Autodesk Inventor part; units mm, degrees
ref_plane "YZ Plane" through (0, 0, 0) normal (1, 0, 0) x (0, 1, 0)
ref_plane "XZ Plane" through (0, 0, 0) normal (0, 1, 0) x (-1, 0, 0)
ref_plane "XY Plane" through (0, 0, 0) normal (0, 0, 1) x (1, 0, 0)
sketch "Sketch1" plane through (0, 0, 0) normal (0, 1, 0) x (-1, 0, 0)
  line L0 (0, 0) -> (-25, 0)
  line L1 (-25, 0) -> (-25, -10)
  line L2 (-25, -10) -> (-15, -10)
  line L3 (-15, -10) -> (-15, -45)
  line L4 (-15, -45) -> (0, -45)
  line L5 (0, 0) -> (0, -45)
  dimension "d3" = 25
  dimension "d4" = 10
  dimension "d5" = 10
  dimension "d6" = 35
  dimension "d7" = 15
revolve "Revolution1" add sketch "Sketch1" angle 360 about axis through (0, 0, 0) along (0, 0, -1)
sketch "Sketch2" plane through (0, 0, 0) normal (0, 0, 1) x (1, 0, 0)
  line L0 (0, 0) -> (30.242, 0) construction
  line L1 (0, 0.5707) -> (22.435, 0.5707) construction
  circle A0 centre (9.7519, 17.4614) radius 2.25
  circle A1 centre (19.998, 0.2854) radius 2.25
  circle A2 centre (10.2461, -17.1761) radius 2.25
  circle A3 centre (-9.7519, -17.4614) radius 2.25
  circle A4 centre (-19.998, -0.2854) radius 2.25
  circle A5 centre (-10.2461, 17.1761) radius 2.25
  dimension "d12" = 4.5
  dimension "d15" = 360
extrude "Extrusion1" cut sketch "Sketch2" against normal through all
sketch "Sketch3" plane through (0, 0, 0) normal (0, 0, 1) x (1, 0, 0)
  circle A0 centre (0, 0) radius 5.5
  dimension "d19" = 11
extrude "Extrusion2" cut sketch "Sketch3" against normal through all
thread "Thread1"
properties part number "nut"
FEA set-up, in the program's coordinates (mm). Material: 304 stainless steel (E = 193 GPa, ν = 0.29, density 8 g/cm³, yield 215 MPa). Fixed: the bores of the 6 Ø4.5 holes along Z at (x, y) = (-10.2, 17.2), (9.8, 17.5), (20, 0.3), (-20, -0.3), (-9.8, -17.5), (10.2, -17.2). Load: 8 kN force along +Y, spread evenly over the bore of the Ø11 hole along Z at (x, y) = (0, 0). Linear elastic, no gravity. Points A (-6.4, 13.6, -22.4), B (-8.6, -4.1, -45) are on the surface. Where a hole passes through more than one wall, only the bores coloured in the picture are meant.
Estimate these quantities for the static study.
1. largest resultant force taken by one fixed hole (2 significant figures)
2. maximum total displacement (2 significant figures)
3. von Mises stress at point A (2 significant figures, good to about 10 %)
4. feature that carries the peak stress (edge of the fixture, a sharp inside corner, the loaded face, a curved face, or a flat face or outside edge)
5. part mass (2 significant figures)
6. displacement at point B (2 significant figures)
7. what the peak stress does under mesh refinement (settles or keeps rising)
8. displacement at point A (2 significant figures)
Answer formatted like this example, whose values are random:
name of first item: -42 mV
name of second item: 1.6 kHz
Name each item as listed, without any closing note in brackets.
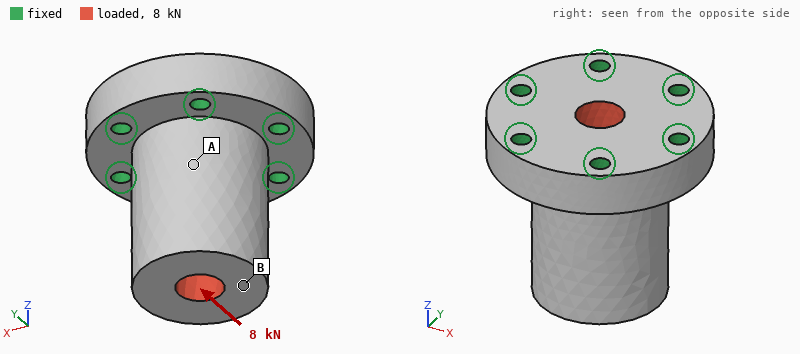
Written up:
largest resultant force taken by one fixed hole: 2.8 kN
maximum total displacement: 14 µm
von Mises stress at point A: 16 MPa
feature that carries the peak stress: edge of the fixture
part mass: 310 g
displacement at point B: 13 µm
what the peak stress does under mesh refinement: keeps rising
displacement at point A: 6.5 µm
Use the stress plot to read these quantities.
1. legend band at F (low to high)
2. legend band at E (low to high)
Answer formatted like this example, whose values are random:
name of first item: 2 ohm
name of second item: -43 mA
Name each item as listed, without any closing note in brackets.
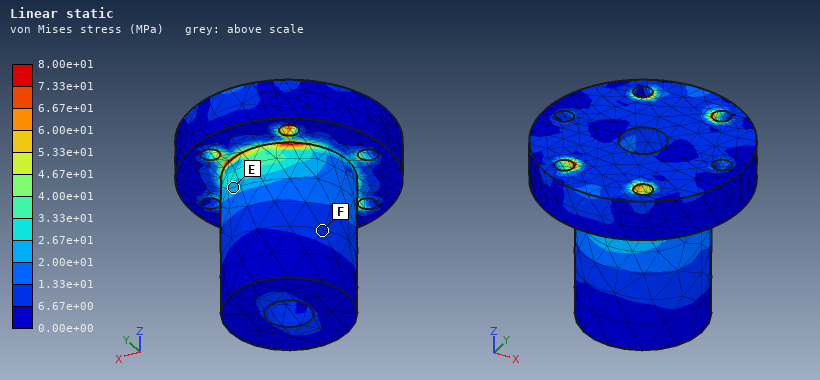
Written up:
legend band at F: 6.67e+00 to 1.33e+01 MPa
legend band at E: 2.00e+01 to 2.67e+01 MPa
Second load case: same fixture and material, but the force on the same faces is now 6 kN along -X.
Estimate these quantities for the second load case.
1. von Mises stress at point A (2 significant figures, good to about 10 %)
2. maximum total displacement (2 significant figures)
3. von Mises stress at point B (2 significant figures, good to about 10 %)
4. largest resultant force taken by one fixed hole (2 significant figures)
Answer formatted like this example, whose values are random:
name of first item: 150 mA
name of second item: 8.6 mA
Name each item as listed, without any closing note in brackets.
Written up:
von Mises stress at point A: 11 MPa
maximum total displacement: 11 µm
von Mises stress at point B: 4.8 MPa
largest resultant force taken by one fixed hole: 2.4 kN
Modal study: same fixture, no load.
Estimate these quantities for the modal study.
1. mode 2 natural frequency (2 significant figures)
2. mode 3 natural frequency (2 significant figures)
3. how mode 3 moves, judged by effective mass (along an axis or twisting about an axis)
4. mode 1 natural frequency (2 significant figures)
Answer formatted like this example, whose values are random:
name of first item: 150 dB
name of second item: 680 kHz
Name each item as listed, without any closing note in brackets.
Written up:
mode 2 natural frequency: 9600 Hz
mode 3 natural frequency: 20 kHz
how mode 3 moves, judged by effective mass: twisting about Z
mode 1 natural frequency: 9600 Hz
